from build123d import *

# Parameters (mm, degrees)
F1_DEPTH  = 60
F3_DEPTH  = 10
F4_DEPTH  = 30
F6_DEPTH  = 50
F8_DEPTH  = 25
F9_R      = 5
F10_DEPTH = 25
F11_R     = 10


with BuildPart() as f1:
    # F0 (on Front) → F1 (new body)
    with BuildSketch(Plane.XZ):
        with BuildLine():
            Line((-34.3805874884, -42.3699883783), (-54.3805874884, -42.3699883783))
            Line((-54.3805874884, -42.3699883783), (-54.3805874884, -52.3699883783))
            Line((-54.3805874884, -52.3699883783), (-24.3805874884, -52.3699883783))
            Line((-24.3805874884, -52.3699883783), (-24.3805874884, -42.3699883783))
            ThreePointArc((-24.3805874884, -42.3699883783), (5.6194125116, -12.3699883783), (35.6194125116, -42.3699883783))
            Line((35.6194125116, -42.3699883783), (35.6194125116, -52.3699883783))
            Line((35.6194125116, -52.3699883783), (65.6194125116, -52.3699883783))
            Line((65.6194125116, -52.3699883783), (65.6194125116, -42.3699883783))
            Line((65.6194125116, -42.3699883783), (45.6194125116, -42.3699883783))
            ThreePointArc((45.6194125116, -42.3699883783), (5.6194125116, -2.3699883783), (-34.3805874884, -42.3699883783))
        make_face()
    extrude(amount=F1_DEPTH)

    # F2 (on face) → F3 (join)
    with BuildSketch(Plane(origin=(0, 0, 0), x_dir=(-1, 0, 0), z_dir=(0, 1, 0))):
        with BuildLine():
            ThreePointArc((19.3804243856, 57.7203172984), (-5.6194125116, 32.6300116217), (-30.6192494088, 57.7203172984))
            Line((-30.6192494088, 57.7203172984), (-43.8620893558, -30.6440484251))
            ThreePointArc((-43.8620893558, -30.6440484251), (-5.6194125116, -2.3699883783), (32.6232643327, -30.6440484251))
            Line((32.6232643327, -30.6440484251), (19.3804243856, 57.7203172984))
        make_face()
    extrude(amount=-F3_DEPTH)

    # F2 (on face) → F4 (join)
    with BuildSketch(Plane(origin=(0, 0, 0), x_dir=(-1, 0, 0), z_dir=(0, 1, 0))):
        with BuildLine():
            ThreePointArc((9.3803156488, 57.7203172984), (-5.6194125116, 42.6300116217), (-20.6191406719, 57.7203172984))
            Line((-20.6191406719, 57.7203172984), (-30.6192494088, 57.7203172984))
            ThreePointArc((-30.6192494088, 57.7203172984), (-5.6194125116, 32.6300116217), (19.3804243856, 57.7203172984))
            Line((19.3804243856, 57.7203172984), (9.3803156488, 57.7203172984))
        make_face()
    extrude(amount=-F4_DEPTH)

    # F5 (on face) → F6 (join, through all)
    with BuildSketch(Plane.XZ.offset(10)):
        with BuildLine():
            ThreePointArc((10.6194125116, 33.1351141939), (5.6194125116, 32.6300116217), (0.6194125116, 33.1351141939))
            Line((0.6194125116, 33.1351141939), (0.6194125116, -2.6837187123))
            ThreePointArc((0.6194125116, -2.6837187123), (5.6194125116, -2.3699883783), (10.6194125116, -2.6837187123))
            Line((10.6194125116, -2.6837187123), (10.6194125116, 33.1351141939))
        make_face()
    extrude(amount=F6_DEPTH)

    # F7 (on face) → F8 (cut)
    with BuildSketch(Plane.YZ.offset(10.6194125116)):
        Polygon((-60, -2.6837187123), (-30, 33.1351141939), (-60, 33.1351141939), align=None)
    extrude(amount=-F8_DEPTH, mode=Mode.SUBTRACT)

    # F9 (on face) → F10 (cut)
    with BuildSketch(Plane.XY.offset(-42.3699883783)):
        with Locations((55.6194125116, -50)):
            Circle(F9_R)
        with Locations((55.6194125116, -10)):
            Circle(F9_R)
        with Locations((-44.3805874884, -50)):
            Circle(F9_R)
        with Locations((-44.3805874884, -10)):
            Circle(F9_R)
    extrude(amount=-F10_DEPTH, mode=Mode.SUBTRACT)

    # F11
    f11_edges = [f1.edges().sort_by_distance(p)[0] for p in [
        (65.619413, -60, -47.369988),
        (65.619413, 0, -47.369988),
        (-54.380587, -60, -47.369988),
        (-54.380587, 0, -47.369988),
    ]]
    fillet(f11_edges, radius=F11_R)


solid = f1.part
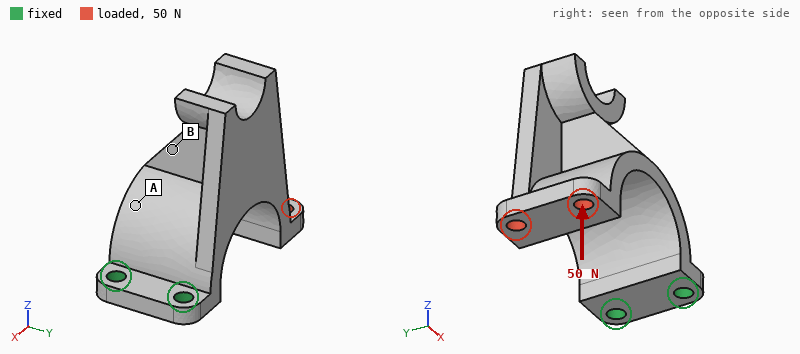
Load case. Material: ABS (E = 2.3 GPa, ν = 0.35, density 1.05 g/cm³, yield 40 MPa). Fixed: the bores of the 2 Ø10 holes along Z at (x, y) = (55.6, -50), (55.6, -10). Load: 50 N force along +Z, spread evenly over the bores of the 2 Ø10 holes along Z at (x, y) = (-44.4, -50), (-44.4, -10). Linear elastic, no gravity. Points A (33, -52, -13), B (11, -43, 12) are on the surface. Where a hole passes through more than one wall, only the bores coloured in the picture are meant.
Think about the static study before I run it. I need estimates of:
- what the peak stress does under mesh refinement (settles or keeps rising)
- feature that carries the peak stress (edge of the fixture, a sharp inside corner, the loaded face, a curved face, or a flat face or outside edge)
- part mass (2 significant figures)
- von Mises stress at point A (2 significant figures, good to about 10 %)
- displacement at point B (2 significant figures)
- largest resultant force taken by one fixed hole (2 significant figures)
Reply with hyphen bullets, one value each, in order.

- keeps rising
- edge of the fixture
- 170 g
- 2.3 MPa
- 0.88 mm
- 26 N
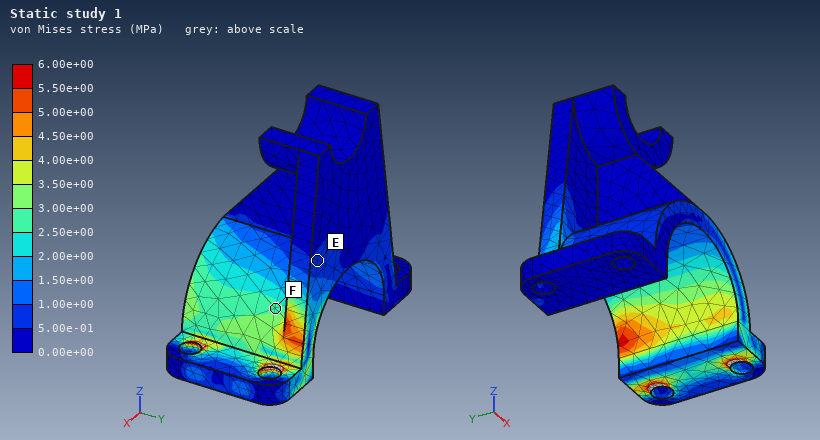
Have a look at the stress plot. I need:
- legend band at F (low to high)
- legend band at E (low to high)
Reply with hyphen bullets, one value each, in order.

- 2.50e+00 to 3.00e+00 MPa
- 5.00e-01 to 1.00e+00 MPa
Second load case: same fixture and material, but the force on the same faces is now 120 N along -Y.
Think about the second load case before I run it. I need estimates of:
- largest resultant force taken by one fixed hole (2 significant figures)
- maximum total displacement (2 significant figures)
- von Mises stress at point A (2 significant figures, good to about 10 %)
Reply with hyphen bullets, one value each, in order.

- 270 N
- 1.9 mm
- 4.8 MPa
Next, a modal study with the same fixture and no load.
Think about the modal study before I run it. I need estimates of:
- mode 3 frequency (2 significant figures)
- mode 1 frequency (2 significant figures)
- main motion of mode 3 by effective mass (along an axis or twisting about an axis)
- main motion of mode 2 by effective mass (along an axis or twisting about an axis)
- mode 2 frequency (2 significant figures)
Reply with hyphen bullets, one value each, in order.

- 450 Hz
- 100 Hz
- along Y
- along Y
- 240 Hz
